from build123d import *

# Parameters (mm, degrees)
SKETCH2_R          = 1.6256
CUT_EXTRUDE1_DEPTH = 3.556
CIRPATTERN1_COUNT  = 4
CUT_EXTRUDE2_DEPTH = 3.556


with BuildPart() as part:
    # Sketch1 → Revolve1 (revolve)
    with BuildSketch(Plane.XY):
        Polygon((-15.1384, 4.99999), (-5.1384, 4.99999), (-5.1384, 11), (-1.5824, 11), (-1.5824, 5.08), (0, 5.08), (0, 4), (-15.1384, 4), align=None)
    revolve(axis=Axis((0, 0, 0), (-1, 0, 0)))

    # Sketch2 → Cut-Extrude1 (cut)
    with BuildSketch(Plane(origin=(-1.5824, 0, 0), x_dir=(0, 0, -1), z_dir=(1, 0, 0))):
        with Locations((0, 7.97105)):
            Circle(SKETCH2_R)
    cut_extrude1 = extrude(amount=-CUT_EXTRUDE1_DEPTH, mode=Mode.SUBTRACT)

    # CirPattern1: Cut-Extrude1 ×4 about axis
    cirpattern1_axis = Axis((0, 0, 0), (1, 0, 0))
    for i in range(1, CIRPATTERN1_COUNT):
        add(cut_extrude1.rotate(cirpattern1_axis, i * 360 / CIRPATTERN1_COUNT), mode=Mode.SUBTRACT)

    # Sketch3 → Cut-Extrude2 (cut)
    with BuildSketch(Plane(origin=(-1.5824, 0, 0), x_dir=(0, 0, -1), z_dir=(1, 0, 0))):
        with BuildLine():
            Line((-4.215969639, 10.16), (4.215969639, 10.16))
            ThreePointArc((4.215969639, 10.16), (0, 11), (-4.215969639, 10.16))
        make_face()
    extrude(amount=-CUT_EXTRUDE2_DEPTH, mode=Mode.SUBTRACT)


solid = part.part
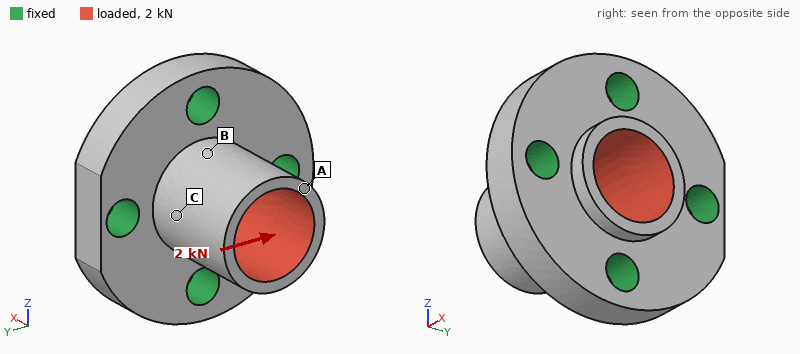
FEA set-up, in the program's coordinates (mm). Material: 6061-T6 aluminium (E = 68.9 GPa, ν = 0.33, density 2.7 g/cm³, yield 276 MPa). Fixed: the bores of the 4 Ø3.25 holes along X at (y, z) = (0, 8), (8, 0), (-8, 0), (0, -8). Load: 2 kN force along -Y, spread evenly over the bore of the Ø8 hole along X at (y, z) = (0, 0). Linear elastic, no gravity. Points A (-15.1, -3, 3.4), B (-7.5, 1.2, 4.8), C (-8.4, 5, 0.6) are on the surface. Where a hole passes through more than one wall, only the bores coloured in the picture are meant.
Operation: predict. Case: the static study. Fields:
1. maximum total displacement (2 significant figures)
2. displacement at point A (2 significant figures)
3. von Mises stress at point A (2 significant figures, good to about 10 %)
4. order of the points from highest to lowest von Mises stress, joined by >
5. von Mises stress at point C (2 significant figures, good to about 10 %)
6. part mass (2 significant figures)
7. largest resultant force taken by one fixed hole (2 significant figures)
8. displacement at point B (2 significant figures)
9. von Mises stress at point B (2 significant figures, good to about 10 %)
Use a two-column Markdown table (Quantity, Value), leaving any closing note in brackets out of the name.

| Quantity | Value |
|---|---|
| maximum total displacement | 39 µm |
| displacement at point A | 37 µm |
| von Mises stress at point A | 20 MPa |
| order of the points from highest to lowest von Mises stress, joined by > | B > C > A |
| von Mises stress at point C | 39 MPa |
| part mass | 3.7 g |
| largest resultant force taken by one fixed hole | 830 N |
| displacement at point B | 12 µm |
| von Mises stress at point B | 94 MPa |
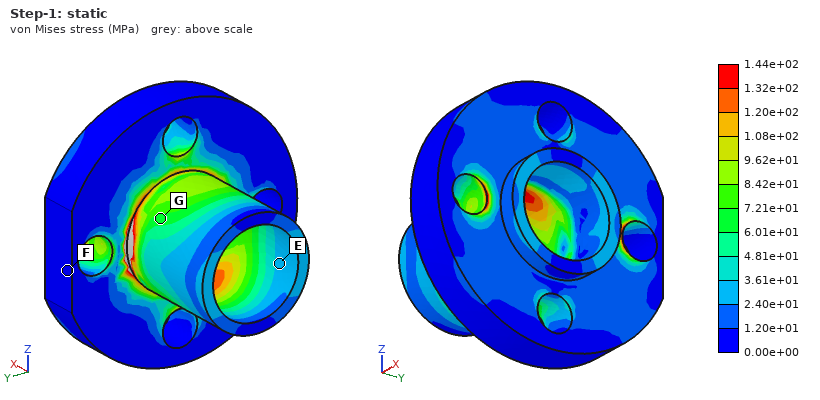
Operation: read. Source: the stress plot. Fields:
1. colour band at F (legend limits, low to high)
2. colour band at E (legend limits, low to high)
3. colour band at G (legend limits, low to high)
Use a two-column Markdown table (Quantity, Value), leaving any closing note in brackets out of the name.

| Quantity | Value |
|---|---|
| colour band at F | 0.00e+00 to 1.20e+01 MPa |
| colour band at E | 2.40e+01 to 3.61e+01 MPa |
| colour band at G | 6.01e+01 to 7.21e+01 MPa |
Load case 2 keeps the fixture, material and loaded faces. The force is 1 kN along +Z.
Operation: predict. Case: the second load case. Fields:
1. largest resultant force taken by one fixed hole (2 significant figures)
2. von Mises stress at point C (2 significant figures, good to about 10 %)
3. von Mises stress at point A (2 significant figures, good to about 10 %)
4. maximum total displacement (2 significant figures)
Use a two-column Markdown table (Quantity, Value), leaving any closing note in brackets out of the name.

| Quantity | Value |
|---|---|
| largest resultant force taken by one fixed hole | 410 N |
| von Mises stress at point C | 46 MPa |
| von Mises stress at point A | 11 MPa |
| maximum total displacement | 19 µm |
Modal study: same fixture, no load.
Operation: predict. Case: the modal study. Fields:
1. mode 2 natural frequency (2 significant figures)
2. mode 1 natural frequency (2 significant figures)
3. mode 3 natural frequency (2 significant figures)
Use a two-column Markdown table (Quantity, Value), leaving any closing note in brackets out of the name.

| Quantity | Value |
|---|---|
| mode 2 natural frequency | 39 kHz |
| mode 1 natural frequency | 39 kHz |
| mode 3 natural frequency | 40 kHz |
